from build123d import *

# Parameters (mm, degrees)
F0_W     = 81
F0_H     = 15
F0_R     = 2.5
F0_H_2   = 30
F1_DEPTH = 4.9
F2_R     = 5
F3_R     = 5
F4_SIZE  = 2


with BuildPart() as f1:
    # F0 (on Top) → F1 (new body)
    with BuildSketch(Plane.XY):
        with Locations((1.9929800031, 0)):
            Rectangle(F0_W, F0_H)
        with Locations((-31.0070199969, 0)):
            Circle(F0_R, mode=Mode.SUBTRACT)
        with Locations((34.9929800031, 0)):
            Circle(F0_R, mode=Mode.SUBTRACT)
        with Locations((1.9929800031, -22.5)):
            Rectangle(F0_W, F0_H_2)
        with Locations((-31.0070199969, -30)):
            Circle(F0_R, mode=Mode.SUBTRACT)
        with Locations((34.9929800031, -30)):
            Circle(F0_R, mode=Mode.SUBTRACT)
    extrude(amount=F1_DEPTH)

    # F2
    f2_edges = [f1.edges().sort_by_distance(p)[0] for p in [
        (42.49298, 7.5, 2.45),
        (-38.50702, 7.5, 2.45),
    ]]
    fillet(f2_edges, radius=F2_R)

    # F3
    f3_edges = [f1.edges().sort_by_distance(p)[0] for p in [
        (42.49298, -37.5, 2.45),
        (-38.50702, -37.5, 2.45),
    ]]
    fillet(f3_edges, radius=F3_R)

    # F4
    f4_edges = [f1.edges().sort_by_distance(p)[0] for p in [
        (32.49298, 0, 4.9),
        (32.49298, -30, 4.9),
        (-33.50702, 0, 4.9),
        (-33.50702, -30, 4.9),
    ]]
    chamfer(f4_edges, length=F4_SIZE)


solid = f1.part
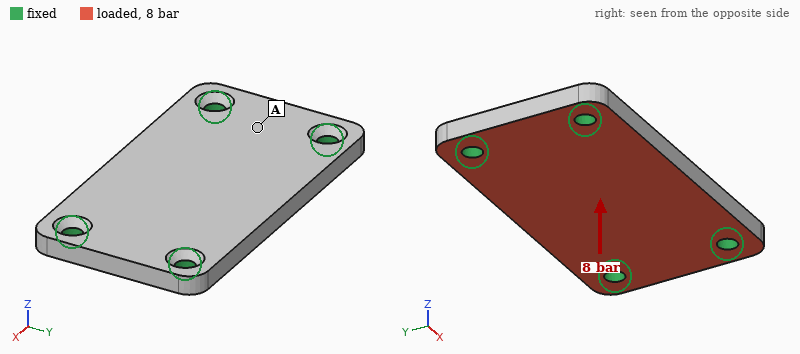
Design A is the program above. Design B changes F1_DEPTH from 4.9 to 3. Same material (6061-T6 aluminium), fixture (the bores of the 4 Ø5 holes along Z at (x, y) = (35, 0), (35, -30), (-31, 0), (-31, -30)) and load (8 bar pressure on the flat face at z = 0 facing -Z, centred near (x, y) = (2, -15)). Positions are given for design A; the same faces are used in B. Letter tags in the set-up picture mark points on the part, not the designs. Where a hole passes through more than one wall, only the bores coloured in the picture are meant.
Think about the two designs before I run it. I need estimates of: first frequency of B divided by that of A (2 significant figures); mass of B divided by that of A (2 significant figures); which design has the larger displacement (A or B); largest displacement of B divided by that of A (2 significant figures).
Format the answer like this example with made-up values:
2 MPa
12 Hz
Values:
0.61
0.61
B
4.4
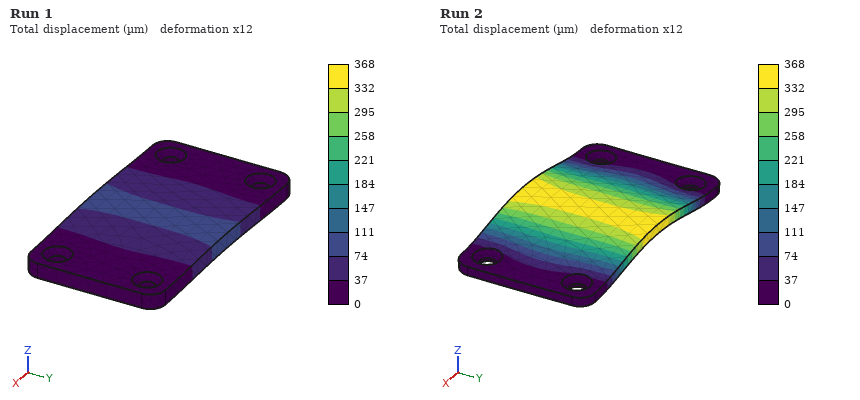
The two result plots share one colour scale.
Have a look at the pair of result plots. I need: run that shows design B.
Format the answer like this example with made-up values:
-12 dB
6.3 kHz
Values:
Run 2
